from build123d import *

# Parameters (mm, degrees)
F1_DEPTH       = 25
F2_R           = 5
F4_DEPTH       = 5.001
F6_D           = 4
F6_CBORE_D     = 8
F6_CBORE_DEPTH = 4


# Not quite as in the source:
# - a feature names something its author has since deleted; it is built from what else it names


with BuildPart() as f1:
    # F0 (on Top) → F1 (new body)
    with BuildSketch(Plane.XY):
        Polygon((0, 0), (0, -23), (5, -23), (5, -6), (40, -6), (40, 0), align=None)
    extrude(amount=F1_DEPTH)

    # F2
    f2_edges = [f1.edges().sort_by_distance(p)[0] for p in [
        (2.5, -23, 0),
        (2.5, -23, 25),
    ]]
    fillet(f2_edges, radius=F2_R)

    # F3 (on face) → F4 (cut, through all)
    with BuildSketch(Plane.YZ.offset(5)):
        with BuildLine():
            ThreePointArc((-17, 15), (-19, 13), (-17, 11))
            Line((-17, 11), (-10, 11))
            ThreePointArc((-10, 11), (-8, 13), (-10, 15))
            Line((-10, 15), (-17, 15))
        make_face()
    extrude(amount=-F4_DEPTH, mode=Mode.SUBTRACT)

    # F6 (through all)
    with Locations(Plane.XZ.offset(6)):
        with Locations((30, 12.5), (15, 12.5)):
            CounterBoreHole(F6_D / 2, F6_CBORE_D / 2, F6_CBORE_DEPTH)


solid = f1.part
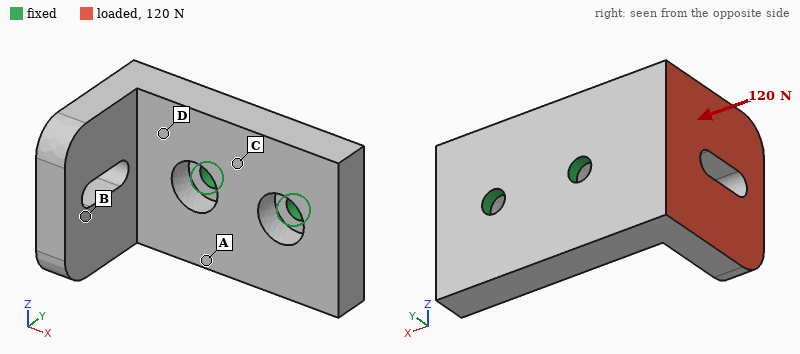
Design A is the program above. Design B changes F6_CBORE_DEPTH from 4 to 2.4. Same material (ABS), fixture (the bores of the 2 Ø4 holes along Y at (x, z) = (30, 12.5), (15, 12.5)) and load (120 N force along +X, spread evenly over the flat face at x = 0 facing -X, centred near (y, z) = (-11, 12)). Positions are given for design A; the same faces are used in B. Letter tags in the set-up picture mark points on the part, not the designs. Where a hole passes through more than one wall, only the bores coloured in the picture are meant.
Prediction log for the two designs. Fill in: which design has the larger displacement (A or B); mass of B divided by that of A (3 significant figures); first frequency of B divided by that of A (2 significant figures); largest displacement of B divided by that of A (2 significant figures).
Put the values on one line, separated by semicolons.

A; 1.02; 1.3; 0.88
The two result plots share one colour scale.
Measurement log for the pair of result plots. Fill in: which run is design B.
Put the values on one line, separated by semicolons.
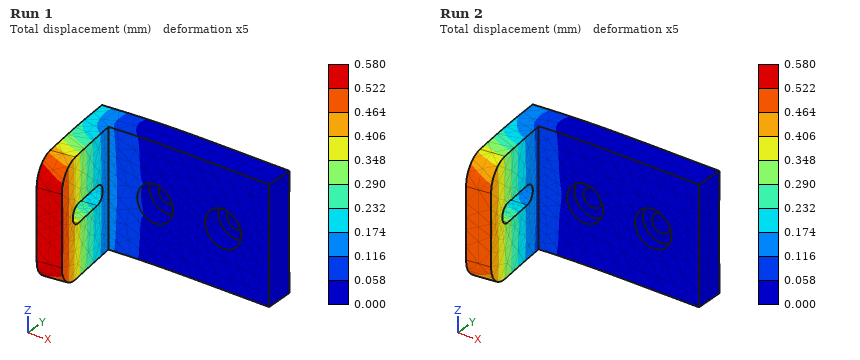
Run 2
